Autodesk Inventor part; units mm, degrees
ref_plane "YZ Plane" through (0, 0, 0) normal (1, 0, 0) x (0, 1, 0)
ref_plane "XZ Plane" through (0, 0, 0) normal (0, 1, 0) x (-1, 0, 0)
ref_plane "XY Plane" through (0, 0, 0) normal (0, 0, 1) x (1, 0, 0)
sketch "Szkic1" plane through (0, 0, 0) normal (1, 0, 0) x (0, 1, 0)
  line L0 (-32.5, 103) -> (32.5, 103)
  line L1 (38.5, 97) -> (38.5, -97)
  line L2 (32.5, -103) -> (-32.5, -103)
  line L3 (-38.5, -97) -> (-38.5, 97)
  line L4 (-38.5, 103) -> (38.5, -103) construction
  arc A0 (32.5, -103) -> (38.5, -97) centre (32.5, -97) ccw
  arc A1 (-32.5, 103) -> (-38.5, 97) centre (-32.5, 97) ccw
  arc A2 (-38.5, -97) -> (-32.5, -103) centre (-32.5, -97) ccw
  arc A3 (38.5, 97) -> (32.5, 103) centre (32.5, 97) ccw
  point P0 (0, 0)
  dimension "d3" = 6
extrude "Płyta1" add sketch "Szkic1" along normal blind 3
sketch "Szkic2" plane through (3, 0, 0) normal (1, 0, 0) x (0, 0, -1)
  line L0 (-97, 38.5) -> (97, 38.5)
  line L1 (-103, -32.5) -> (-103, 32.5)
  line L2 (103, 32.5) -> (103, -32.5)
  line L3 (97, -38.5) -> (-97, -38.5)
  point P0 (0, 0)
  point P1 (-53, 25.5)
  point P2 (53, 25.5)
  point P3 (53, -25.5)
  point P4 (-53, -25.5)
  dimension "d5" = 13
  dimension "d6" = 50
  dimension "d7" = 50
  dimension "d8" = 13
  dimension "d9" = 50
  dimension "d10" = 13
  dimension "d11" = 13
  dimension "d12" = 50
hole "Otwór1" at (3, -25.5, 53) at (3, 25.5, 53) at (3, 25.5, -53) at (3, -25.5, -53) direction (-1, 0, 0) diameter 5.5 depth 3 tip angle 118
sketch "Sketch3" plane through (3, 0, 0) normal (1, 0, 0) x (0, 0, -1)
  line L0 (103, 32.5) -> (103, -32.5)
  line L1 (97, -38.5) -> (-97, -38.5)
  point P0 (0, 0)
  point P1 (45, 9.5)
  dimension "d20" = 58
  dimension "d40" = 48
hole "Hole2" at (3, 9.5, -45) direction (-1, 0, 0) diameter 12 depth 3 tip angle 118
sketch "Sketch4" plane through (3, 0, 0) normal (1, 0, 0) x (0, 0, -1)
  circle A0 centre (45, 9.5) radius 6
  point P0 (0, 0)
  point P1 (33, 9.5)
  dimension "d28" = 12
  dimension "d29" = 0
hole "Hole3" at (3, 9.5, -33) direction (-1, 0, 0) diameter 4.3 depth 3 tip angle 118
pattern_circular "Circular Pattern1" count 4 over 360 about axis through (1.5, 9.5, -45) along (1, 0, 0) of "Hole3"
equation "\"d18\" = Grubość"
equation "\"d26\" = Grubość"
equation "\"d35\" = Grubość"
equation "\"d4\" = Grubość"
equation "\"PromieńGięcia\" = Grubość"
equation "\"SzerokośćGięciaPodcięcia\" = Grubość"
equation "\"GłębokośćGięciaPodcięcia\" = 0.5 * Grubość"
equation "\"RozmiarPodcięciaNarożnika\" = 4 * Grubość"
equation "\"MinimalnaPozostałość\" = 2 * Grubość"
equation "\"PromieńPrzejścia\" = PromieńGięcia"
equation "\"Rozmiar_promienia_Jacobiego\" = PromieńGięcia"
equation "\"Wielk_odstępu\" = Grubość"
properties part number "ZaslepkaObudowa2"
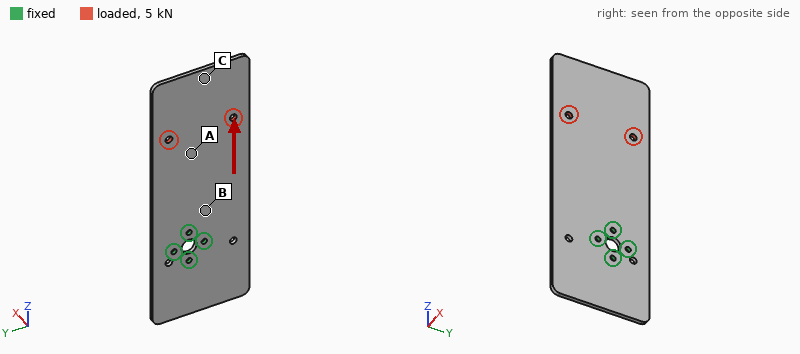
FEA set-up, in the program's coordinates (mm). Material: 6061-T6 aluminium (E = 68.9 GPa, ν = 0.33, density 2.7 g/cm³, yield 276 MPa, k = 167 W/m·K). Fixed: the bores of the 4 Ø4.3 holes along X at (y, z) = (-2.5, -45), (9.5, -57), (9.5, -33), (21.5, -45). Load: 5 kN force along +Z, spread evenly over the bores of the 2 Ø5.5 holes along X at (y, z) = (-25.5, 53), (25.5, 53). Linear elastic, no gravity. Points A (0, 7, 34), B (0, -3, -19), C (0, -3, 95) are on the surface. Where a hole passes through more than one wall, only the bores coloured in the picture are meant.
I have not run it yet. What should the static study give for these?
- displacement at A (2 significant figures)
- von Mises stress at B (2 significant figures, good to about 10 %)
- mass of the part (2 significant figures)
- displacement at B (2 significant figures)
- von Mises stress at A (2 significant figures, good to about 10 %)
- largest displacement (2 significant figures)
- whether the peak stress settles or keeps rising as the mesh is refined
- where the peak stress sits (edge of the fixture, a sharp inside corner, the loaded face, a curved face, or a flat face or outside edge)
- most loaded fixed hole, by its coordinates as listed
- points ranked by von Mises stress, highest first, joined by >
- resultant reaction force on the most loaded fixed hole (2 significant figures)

39 µm
28 MPa
130 g
16 µm
18 MPa
76 µm
keeps rising
edge of the fixture
(-2.5, -45)
B > A > C
2.5 kN
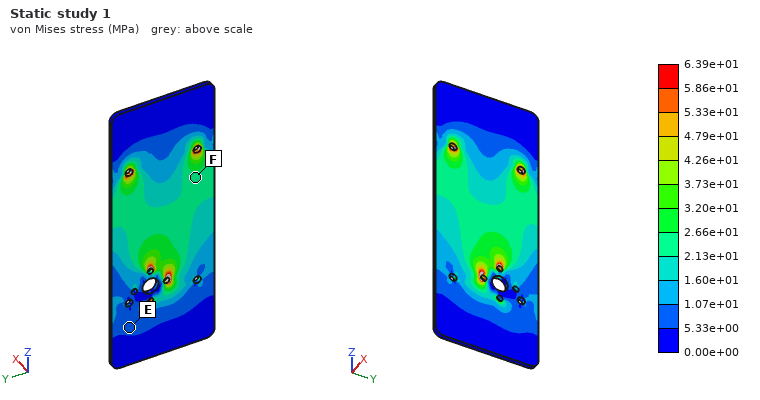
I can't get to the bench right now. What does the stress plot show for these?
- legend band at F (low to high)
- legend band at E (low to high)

2.13e+01 to 2.66e+01 MPa
5.33e+00 to 1.07e+01 MPa
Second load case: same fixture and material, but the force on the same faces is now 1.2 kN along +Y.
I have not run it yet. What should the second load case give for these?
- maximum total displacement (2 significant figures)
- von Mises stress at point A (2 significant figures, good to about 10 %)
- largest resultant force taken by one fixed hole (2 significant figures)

0.21 mm
13 MPa
2.6 kN
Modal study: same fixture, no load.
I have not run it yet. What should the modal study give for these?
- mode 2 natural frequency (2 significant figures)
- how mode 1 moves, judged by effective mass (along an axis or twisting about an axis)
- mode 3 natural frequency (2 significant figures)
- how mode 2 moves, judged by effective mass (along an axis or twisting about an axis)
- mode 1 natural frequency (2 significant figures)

440 Hz
along X
760 Hz
twisting about Z
130 Hz
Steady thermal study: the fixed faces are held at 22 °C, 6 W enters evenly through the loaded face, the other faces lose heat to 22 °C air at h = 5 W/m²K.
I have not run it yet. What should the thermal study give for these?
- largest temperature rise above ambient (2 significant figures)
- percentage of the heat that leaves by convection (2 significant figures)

14 K
17 %
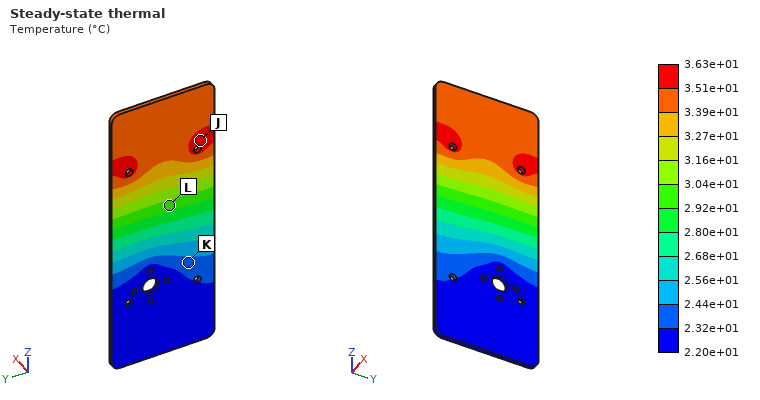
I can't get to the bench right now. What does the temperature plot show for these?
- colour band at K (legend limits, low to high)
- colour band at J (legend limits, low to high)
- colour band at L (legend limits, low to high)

2.32e+01 to 2.44e+01 °C
3.51e+01 to 3.63e+01 °C
2.92e+01 to 3.04e+01 °C
